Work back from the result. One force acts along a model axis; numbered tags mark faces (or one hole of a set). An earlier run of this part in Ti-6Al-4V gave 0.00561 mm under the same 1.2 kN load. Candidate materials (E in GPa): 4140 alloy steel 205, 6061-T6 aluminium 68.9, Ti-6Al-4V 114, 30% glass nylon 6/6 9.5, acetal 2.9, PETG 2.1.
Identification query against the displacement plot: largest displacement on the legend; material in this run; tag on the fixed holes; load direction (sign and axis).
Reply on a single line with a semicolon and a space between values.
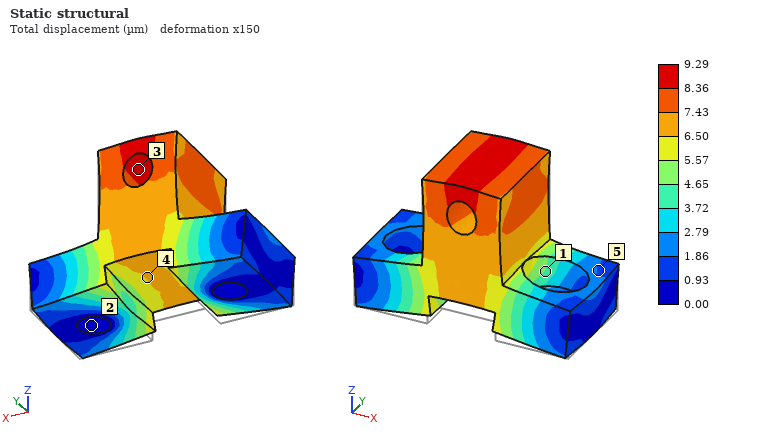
9.29 µm; 6061-T6 aluminium; 2; +Z
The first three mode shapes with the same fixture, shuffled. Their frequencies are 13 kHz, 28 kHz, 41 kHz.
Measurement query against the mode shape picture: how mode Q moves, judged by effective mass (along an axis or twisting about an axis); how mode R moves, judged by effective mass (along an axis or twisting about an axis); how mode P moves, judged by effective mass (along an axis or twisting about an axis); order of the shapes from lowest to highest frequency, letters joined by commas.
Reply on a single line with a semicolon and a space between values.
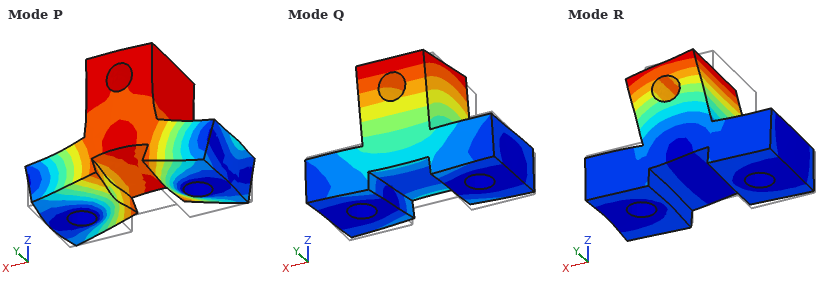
along Y; along X; along Z; Q, R, P
